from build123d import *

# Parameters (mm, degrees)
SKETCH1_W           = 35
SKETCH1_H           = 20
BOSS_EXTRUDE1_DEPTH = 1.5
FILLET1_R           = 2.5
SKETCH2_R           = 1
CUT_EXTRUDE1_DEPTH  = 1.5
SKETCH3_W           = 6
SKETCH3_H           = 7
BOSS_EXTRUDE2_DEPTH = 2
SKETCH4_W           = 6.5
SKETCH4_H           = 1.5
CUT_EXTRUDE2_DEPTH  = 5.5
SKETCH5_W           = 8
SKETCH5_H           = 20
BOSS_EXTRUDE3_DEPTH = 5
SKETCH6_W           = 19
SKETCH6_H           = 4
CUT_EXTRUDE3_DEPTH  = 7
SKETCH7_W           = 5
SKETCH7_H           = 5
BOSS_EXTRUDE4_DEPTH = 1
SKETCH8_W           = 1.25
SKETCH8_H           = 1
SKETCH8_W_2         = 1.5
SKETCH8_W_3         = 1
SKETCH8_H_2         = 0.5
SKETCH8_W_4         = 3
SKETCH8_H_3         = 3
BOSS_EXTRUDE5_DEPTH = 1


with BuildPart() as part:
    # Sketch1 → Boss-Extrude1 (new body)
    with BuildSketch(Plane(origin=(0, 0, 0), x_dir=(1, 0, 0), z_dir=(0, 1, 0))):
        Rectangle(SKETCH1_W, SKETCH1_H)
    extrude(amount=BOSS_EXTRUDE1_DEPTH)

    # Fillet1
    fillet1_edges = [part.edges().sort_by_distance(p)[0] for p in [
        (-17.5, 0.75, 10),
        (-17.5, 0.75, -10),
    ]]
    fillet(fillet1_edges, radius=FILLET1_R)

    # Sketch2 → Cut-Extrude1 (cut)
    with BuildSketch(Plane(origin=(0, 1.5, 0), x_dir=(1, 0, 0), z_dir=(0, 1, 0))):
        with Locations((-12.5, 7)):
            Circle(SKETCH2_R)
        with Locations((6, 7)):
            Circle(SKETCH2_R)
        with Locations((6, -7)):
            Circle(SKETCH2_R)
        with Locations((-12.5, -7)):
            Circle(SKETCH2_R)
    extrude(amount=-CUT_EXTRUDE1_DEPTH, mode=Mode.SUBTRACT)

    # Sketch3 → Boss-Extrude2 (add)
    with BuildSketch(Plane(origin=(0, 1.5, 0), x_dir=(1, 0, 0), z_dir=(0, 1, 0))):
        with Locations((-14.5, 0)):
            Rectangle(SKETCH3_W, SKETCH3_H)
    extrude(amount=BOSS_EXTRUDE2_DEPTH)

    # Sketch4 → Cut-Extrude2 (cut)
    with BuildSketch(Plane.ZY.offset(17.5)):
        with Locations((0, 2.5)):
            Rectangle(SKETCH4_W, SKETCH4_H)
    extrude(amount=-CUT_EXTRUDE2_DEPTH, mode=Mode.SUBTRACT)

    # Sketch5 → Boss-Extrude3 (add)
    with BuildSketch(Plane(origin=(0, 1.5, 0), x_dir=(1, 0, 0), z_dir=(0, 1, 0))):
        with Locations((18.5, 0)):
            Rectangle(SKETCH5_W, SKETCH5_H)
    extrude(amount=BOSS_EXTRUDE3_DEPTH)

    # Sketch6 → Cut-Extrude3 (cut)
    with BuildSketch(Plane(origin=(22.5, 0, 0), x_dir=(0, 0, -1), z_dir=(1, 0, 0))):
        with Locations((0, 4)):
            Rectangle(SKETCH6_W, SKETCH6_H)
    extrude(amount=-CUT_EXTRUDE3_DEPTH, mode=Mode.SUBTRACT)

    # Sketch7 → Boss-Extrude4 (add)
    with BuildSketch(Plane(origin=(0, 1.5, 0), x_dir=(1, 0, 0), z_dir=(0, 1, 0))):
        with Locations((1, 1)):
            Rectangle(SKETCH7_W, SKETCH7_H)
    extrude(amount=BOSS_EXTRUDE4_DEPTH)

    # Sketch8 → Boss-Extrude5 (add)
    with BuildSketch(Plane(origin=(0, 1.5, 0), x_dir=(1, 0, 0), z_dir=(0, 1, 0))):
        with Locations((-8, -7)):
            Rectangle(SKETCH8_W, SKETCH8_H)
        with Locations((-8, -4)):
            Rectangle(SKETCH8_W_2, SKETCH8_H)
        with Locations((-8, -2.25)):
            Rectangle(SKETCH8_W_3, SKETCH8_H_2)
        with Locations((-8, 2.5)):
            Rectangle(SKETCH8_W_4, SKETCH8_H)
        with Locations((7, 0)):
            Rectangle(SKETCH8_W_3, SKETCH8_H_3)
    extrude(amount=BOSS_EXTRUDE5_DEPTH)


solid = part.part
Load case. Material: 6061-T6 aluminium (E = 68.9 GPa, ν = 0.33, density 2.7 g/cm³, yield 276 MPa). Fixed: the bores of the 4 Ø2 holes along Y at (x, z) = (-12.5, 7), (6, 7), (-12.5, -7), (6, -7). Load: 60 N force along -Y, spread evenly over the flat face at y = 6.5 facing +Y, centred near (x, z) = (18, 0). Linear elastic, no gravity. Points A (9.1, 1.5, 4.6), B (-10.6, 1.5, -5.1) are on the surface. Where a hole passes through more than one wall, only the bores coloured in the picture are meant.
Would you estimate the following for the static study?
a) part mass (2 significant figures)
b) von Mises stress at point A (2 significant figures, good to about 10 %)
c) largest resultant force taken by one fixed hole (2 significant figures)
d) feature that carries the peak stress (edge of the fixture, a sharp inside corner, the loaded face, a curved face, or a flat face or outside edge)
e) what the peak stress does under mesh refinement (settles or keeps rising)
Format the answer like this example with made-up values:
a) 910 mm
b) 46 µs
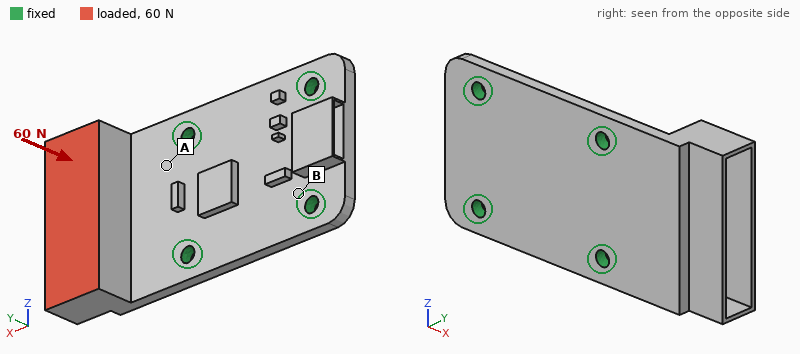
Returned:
a) 3.7 g
b) 66 MPa
c) 34 N
d) edge of the fixture
e) keeps rising
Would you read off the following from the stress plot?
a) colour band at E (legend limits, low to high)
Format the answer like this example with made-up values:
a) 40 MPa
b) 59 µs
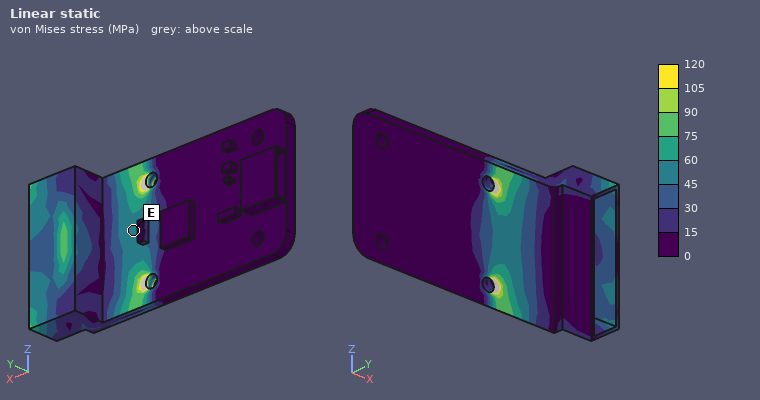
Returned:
a) 45 to 60 MPa
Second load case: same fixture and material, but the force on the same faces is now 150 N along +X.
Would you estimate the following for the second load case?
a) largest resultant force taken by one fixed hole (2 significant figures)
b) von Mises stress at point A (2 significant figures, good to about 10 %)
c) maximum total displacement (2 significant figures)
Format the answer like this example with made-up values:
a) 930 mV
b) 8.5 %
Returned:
a) 65 N
b) 110 MPa
c) 0.32 mm
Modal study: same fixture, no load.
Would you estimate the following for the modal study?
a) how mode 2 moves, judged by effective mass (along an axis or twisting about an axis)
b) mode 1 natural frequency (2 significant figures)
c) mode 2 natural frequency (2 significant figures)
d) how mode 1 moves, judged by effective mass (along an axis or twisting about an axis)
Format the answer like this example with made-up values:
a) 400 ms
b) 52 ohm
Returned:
a) twisting about X
b) 4100 Hz
c) 8100 Hz
d) along Y
